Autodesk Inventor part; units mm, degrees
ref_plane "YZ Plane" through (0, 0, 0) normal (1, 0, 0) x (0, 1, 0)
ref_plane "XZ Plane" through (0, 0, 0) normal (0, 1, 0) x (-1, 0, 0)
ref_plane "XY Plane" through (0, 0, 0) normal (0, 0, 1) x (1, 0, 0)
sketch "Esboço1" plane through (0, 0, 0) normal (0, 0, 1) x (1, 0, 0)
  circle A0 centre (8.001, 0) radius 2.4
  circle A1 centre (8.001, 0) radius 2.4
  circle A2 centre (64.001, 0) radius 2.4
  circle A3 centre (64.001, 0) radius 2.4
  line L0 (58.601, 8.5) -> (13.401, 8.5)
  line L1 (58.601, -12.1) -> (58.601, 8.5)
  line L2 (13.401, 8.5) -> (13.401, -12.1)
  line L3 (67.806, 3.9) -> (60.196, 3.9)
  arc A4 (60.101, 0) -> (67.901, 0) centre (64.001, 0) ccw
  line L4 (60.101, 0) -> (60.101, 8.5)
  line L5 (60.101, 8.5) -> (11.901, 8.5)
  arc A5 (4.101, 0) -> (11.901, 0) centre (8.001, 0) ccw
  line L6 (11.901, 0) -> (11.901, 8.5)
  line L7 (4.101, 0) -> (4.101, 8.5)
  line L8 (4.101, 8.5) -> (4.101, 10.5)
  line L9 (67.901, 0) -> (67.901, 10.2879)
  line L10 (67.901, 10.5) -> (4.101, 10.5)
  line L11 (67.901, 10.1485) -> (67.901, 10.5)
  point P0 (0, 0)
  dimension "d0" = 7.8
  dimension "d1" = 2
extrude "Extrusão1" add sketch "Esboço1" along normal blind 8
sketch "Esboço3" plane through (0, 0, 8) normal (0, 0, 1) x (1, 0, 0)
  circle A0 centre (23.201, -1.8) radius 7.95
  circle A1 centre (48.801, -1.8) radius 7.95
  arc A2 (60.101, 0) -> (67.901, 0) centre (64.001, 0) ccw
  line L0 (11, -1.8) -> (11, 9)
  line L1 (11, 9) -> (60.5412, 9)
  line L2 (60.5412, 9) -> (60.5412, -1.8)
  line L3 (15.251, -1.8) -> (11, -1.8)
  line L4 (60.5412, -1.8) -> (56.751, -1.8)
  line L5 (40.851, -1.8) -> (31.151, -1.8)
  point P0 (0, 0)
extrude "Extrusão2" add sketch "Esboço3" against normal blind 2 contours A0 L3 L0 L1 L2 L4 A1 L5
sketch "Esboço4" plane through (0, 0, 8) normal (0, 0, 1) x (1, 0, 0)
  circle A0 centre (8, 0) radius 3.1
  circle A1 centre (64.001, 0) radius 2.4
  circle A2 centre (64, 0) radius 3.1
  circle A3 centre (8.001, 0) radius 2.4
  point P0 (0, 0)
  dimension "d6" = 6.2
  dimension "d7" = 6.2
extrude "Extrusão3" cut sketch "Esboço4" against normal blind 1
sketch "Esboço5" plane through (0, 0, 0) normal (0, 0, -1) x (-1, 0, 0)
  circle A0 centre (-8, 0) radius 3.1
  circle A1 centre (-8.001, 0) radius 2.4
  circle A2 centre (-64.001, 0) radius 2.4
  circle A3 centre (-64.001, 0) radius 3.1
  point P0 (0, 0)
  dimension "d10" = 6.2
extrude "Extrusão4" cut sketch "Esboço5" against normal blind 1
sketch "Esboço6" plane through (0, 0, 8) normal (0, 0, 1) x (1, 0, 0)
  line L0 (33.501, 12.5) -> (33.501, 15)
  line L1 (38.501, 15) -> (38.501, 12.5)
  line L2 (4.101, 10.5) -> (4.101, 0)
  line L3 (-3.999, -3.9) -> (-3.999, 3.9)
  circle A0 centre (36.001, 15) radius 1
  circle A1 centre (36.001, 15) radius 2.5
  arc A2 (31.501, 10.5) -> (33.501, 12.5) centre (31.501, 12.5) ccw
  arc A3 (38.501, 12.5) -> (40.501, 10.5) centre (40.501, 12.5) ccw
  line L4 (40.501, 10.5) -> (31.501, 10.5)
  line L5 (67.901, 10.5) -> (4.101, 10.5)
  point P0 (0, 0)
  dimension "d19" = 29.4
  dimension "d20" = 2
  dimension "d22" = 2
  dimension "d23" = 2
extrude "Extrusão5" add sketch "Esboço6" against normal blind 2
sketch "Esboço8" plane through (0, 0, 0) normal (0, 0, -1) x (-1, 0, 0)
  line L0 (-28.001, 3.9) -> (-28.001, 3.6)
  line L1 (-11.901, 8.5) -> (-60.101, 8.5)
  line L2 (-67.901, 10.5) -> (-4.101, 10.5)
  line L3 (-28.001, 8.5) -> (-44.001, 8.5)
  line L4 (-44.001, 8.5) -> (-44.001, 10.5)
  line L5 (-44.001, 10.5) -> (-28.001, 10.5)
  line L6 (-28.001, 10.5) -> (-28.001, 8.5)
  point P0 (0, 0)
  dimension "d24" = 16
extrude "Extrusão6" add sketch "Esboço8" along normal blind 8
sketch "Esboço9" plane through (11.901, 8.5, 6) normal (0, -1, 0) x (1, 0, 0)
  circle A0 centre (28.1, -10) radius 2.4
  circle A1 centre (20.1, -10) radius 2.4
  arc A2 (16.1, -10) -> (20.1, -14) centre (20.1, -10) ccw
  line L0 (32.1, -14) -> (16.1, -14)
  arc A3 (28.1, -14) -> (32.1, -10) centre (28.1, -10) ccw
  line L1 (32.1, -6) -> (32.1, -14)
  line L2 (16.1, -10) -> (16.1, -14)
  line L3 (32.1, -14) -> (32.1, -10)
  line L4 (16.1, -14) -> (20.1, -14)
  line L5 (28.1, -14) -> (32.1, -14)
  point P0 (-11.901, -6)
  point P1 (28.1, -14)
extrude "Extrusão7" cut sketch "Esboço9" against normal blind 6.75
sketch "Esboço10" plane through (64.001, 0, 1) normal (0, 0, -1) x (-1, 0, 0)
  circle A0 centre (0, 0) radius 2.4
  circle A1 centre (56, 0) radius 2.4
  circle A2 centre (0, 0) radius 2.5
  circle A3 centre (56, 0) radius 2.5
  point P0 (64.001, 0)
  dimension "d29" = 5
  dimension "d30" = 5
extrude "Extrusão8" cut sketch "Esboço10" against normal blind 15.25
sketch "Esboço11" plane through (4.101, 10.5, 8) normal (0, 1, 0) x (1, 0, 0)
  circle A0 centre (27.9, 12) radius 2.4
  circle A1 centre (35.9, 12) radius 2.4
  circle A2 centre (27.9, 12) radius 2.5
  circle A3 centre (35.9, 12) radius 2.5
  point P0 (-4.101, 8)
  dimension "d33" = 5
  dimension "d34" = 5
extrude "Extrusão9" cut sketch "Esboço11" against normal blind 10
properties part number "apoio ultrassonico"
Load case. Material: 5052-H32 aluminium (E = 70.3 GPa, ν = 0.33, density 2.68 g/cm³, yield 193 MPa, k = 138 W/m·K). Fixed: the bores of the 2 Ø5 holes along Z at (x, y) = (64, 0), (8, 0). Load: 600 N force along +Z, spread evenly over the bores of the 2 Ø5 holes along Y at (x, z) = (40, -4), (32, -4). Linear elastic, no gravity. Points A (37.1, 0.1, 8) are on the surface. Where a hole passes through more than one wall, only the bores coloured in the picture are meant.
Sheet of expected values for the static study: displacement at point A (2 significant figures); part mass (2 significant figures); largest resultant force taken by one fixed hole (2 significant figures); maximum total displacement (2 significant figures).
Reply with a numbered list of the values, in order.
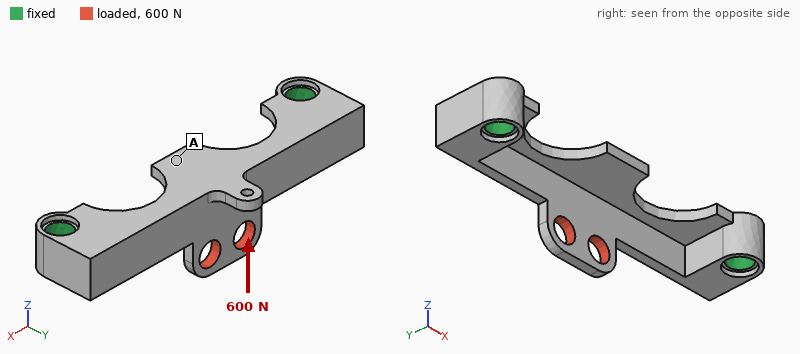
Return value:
1. 71 µm
2. 7.9 g
3. 300 N
4. 96 µm
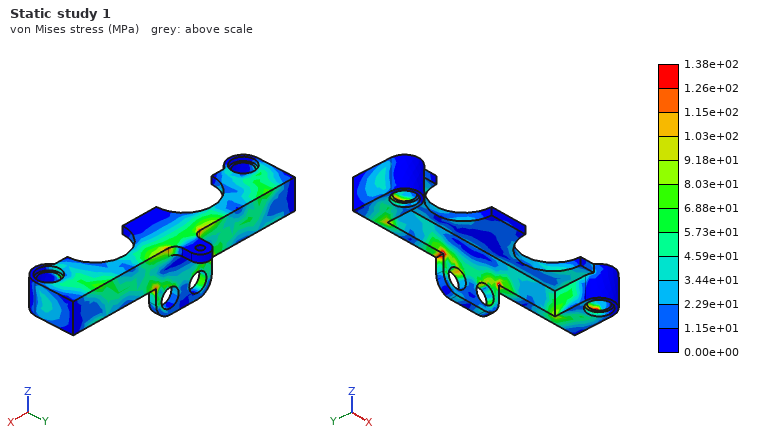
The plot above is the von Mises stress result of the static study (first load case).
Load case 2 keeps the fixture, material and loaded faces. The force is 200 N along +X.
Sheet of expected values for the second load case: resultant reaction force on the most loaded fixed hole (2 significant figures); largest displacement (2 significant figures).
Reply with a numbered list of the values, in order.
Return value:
1. 110 N
2. 15 µm
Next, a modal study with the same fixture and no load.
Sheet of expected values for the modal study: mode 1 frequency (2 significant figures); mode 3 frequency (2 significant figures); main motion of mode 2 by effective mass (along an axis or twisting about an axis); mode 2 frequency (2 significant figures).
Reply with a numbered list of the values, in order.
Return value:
1. 4800 Hz
2. 13 kHz
3. along Z
4. 7500 Hz
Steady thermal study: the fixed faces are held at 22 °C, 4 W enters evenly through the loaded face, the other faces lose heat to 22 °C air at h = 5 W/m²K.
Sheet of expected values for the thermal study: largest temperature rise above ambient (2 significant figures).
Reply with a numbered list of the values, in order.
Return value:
1. 23 K
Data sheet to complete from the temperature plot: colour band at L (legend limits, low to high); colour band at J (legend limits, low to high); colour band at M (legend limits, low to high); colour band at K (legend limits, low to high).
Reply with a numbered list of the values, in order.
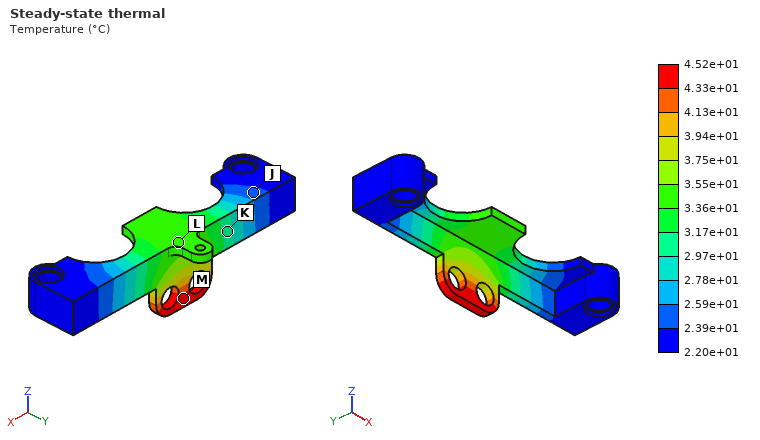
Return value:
1. 3.36e+01 to 3.55e+01 °C
2. 2.39e+01 to 2.59e+01 °C
3. 4.33e+01 to 4.52e+01 °C
4. 2.97e+01 to 3.17e+01 °C
